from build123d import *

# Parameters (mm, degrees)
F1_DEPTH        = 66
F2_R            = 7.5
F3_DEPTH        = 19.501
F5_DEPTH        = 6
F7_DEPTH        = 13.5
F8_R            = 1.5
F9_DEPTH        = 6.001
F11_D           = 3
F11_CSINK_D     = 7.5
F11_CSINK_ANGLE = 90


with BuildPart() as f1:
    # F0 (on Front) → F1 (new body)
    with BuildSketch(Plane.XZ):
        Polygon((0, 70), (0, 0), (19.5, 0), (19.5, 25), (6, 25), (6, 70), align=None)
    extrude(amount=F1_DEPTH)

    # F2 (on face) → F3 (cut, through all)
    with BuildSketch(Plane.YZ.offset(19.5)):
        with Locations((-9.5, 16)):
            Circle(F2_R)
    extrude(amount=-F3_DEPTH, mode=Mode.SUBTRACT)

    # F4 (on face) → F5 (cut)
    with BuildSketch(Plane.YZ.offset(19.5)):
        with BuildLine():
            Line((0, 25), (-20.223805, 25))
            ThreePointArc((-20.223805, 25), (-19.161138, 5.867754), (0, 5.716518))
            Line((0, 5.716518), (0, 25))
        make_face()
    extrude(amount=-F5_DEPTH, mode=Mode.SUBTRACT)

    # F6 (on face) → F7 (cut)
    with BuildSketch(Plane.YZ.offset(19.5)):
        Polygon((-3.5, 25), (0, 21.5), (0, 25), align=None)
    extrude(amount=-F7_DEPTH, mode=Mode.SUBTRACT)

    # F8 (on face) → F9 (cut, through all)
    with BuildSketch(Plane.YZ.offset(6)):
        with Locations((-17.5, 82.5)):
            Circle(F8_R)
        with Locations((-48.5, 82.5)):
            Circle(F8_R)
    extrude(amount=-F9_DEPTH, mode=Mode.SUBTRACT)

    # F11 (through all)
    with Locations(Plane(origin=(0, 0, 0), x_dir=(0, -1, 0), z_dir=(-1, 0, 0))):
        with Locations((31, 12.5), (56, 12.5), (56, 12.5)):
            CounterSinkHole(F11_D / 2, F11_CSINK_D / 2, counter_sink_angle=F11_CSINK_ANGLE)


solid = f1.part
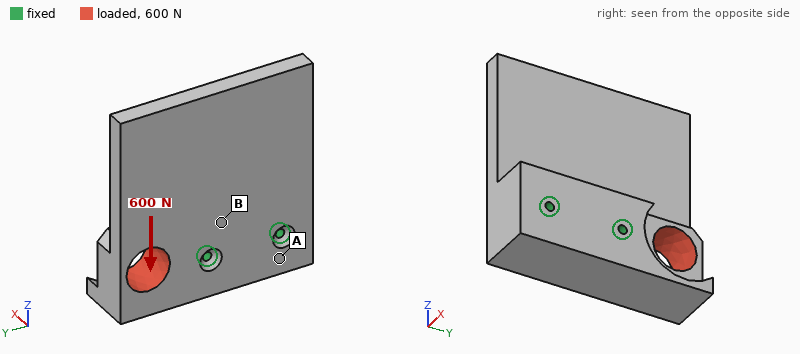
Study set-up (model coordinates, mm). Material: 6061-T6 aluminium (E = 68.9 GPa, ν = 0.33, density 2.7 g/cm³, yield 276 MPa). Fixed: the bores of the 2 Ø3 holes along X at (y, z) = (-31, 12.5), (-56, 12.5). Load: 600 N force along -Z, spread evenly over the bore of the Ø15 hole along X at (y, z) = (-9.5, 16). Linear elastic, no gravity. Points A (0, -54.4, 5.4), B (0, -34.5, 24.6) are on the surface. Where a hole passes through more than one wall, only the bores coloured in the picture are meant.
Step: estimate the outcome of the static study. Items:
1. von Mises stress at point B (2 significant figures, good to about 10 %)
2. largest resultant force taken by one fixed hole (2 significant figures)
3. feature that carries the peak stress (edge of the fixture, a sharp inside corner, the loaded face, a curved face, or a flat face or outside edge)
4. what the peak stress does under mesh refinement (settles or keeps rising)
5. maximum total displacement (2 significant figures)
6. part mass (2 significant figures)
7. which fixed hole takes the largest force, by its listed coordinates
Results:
2.5 MPa
1.1 kN
edge of the fixture
keeps rising
7.1 µm
120 g
(-31, 12.5)
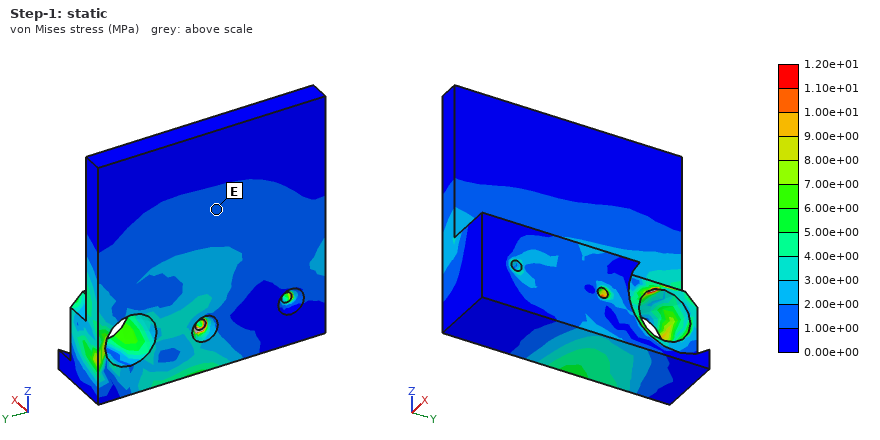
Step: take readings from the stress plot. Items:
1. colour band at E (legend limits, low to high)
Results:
1.00e+00 to 2.00e+00 MPa
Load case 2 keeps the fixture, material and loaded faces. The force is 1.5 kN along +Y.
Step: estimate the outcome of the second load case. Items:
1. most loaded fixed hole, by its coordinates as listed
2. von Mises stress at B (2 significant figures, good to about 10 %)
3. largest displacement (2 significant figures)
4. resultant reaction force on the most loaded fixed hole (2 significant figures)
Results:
(-31, 12.5)
3.4 MPa
7.2 µm
1.1 kN
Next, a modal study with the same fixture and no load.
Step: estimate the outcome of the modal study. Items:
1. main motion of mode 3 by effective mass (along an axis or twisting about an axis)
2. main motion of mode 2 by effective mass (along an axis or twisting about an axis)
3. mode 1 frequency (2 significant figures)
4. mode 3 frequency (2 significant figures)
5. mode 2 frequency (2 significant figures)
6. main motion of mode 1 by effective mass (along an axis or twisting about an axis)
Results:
along Y
twisting about Z
2000 Hz
6500 Hz
3600 Hz
along X
